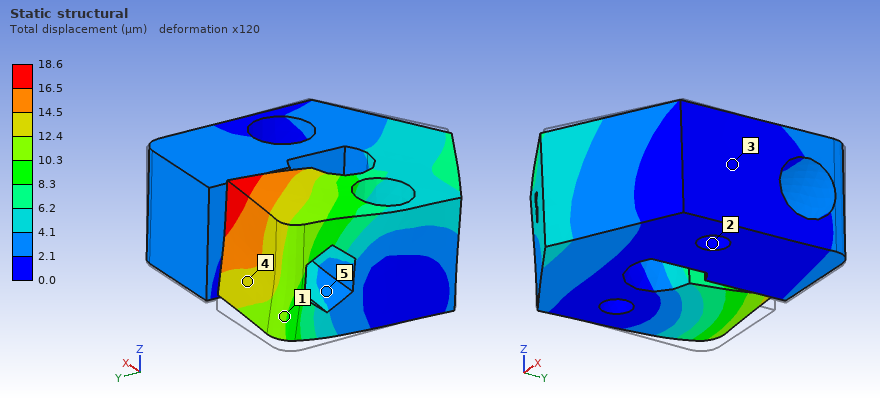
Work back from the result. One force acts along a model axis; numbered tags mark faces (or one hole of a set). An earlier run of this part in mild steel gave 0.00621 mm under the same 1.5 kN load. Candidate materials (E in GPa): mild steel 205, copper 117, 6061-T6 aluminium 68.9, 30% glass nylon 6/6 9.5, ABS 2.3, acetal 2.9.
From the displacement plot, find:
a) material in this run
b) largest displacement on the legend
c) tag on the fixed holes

6061-T6 aluminium
18.6 µm
2
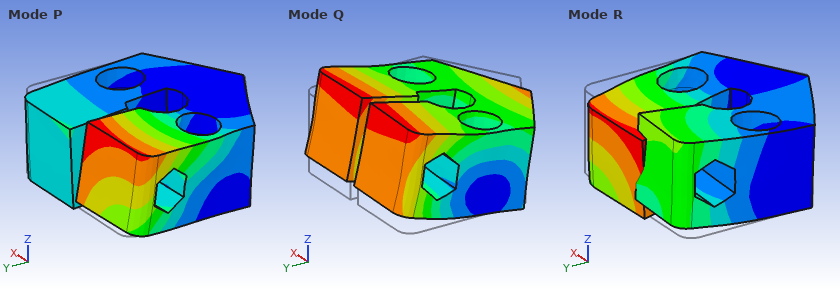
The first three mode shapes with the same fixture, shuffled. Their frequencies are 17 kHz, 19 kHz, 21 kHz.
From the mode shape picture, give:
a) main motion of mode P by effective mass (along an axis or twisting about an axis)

along X
